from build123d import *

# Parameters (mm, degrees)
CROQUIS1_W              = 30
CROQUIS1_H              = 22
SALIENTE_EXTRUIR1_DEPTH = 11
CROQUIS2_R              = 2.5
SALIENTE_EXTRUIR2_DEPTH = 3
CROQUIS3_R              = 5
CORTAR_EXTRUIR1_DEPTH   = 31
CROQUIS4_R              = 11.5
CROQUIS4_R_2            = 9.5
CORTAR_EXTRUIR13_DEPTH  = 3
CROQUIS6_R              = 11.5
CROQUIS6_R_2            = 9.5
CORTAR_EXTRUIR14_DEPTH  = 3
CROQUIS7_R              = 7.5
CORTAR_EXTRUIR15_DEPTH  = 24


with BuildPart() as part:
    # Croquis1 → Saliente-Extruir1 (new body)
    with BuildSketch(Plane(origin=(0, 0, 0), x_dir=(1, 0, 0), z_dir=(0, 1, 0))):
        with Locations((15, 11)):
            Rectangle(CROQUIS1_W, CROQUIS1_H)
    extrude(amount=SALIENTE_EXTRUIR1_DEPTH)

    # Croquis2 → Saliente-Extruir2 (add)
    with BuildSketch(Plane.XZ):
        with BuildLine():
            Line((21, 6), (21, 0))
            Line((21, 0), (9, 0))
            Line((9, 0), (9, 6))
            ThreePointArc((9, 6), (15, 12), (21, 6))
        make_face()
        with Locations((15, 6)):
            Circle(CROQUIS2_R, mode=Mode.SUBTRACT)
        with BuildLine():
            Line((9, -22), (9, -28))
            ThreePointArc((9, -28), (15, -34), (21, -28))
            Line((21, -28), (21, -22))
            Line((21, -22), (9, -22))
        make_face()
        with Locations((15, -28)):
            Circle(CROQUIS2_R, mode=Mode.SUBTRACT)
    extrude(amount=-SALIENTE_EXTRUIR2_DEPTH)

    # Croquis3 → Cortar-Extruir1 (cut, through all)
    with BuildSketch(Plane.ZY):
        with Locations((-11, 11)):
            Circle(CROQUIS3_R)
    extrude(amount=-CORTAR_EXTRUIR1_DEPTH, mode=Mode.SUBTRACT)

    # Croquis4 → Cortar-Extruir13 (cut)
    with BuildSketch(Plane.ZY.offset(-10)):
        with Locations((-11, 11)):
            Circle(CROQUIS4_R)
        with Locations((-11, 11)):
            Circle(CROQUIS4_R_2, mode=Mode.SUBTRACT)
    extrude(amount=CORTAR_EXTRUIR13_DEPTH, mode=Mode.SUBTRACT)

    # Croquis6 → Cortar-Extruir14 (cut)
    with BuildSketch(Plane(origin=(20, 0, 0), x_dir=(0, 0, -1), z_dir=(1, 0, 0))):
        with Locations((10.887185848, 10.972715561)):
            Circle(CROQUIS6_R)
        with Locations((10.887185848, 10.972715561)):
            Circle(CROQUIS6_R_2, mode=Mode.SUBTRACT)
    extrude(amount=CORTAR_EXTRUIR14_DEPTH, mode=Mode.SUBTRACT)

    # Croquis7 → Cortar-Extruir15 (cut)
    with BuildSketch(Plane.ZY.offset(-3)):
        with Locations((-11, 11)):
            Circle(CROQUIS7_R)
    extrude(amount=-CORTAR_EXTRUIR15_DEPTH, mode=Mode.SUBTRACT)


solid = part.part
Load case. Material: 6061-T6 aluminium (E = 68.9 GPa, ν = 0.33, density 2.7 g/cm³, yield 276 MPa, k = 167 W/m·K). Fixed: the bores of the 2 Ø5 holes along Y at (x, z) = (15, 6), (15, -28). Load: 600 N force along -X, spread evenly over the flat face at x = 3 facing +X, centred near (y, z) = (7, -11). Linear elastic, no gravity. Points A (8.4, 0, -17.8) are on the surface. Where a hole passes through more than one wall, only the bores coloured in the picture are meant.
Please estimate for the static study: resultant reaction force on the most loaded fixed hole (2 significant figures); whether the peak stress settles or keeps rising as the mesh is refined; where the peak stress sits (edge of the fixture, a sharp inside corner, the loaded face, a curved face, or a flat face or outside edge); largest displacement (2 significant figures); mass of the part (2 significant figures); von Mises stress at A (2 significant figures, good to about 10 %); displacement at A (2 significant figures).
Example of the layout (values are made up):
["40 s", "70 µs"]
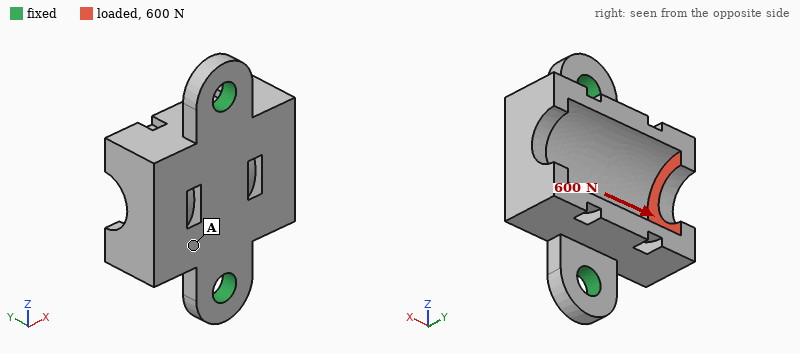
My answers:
["300 N", "keeps rising", "edge of the fixture", "51 µm", "14 g", "15 MPa", "16 µm"]
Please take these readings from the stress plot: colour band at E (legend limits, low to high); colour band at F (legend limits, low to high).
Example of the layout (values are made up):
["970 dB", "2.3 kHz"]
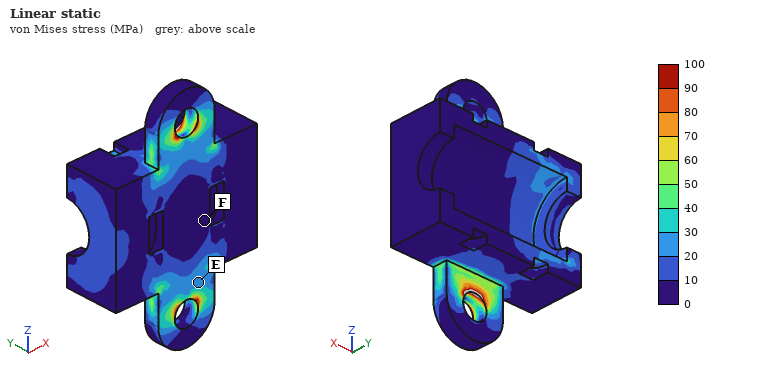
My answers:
["20 to 30 MPa", "0 to 10 MPa"]
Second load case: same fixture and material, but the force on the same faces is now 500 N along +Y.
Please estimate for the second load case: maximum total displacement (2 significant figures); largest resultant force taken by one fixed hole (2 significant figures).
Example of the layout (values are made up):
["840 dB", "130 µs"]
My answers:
["92 µm", "290 N"]
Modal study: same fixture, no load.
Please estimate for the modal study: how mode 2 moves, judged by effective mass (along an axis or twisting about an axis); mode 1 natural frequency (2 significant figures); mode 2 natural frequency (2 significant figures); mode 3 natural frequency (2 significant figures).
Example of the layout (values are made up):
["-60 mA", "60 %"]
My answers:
["along Y", "5200 Hz", "11 kHz", "17 kHz"]
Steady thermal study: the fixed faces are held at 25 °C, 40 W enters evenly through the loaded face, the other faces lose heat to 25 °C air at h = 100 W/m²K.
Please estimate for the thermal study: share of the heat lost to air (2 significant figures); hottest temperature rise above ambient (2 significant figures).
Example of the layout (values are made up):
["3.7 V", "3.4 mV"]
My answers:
["18 %", "51 K"]
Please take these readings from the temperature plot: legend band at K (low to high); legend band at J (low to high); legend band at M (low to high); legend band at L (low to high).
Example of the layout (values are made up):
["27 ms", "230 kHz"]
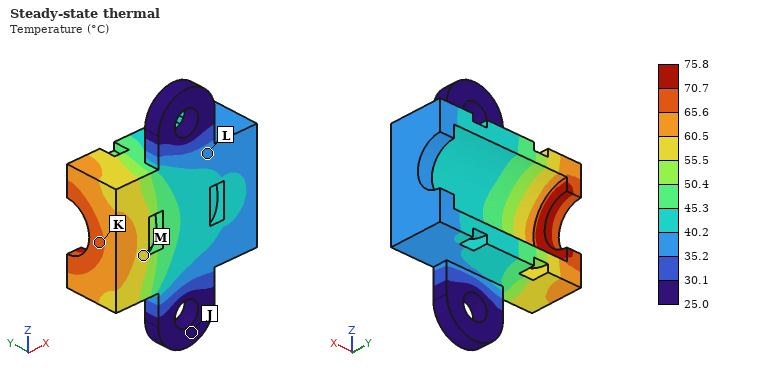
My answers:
["65.6 to 70.7 °C", "25.0 to 30.1 °C", "55.5 to 60.5 °C", "35.2 to 40.2 °C"]
